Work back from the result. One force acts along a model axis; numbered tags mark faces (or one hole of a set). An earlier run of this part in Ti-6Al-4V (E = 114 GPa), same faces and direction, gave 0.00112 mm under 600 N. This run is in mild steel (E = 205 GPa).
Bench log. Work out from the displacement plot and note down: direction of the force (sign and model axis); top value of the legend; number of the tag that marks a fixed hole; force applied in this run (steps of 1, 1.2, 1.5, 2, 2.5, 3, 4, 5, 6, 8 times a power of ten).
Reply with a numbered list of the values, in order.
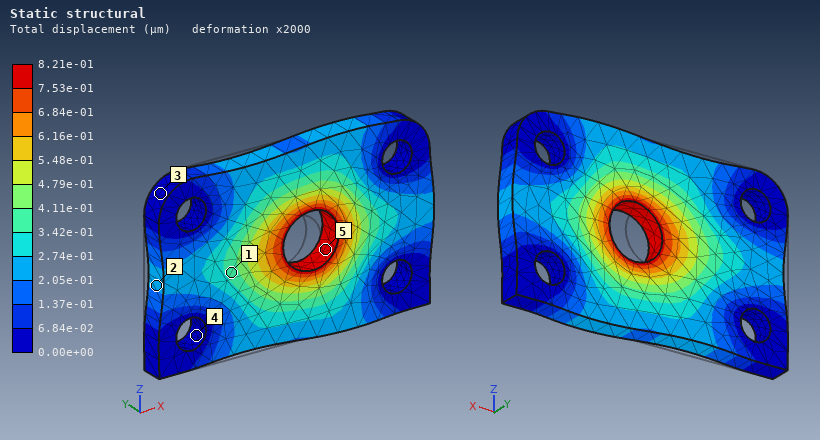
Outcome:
1. +X
2. 8.21e-01 µm
3. 4
4. 800 N
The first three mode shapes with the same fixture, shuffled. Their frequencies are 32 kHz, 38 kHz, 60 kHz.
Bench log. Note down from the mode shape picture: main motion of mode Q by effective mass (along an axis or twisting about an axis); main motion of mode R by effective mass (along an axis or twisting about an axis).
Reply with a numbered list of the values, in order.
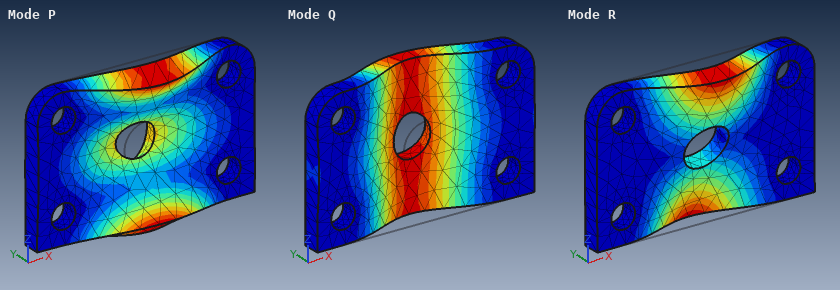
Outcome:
1. along Y
2. twisting about X
